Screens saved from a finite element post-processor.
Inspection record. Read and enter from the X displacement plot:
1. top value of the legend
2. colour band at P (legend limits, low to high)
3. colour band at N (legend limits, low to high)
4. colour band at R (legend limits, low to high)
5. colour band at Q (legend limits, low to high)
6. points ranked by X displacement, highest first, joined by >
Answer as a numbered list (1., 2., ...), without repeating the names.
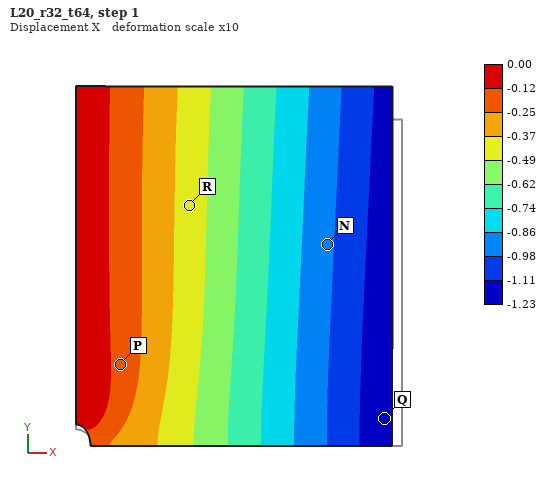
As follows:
1. 0.00
2. -0.25 to -0.12
3. -0.98 to -0.86
4. -0.49 to -0.37
5. -1.23 to -1.11
6. P > R > N > Q
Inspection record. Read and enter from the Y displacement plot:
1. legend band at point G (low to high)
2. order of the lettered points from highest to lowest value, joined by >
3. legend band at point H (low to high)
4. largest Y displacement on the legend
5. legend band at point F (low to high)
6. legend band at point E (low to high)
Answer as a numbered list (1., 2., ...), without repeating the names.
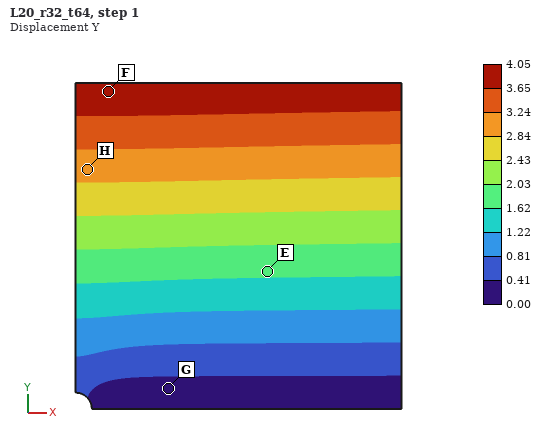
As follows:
1. 0.00 to 0.41
2. F > H > E > G
3. 2.84 to 3.24
4. 4.05
5. 3.65 to 4.05
6. 1.62 to 2.03
